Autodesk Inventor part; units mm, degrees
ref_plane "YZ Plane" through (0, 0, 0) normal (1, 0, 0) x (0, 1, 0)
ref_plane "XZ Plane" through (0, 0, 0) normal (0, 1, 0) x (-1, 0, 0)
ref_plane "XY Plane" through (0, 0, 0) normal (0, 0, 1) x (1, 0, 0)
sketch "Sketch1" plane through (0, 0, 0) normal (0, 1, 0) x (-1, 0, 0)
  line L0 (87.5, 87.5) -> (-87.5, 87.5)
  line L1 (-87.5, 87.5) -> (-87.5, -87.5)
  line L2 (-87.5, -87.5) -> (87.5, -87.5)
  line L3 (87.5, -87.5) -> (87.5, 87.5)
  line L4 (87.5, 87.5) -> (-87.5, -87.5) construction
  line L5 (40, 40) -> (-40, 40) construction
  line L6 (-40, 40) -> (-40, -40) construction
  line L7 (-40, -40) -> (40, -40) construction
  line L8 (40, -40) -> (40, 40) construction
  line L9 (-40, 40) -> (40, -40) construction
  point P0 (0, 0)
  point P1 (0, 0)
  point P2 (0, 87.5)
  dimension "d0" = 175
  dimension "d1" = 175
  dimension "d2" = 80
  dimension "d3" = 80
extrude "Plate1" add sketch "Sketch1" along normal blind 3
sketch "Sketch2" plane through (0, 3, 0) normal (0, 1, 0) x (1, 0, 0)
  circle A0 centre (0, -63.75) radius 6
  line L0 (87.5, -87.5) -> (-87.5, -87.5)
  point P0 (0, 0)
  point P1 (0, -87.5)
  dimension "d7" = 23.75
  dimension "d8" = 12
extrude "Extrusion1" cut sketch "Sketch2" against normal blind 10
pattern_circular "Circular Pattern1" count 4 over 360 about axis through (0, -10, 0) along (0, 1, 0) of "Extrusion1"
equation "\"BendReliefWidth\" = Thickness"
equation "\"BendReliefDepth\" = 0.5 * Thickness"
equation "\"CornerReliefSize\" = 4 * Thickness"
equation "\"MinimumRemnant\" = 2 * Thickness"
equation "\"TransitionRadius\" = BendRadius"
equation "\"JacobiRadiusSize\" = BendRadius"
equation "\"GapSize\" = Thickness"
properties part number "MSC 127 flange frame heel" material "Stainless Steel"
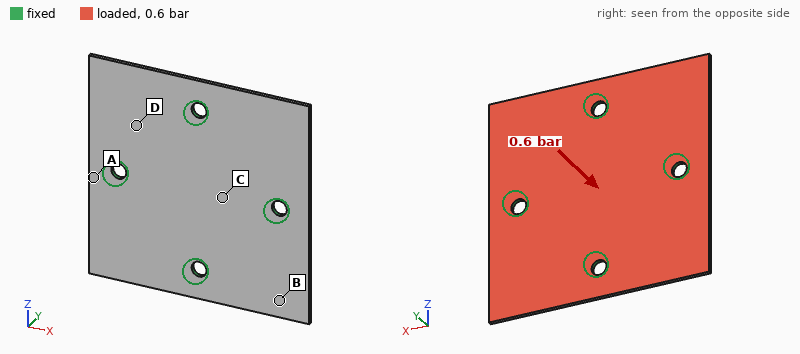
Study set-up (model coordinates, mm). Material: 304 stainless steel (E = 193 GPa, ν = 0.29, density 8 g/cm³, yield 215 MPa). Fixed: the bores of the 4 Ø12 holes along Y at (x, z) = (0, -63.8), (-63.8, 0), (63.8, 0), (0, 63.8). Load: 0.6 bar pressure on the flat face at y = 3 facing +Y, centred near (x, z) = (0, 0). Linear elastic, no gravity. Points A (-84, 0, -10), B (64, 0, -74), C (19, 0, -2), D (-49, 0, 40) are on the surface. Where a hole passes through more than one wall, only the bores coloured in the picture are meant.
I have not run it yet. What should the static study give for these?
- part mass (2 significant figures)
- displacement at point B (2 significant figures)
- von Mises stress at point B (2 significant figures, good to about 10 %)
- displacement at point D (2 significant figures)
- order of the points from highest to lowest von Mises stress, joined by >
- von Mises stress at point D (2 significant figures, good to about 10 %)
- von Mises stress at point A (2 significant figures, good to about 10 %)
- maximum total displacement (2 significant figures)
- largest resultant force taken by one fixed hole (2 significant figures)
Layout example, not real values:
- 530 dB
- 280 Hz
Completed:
- 720 g
- 0.17 mm
- 17 MPa
- 0.056 mm
- A > D > B > C
- 27 MPa
- 43 MPa
- 0.28 mm
- 450 N
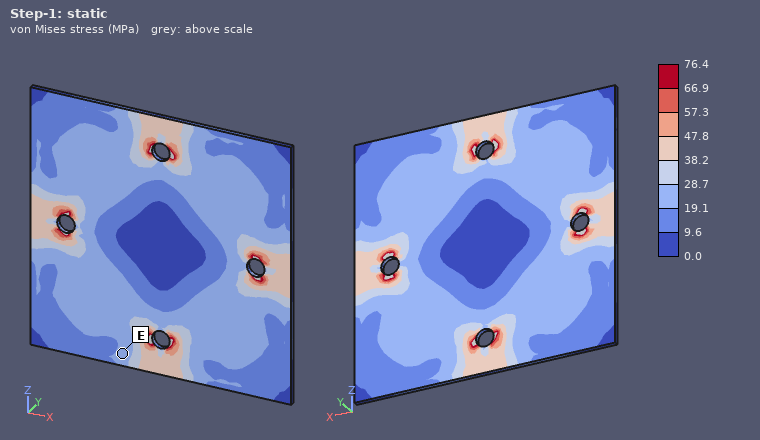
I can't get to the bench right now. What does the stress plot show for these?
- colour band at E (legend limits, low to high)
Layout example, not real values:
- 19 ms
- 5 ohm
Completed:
- 19.1 to 28.7 MPa
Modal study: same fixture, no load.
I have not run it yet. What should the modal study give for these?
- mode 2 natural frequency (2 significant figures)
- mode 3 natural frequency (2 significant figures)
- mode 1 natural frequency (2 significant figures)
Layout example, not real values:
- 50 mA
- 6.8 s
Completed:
- 660 Hz
- 660 Hz
- 650 Hz
